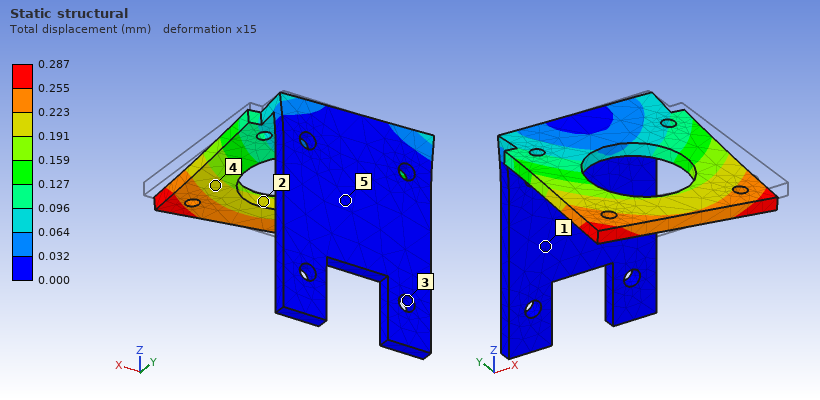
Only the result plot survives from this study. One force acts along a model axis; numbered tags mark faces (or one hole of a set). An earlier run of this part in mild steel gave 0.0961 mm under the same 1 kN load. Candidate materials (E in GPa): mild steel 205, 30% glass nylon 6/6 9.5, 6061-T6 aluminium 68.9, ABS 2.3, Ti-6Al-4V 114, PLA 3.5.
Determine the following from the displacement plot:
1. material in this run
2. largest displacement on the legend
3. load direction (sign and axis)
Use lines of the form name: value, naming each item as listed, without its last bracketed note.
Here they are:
material in this run: 6061-T6 aluminium
largest displacement on the legend: 0.287 mm
load direction: -X
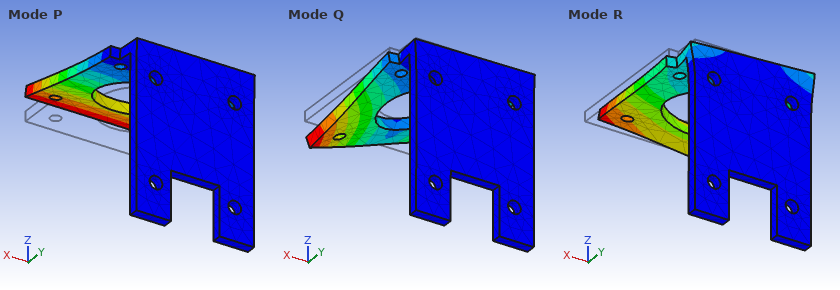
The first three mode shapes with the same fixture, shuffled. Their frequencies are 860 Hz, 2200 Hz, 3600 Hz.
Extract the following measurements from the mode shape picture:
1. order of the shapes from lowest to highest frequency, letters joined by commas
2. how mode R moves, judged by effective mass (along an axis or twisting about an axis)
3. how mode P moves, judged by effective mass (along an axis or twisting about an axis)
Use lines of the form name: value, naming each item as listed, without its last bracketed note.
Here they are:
order of the shapes from lowest to highest frequency, letters joined by commas: P, Q, R
how mode R moves, judged by effective mass: along X
how mode P moves, judged by effective mass: along Z
